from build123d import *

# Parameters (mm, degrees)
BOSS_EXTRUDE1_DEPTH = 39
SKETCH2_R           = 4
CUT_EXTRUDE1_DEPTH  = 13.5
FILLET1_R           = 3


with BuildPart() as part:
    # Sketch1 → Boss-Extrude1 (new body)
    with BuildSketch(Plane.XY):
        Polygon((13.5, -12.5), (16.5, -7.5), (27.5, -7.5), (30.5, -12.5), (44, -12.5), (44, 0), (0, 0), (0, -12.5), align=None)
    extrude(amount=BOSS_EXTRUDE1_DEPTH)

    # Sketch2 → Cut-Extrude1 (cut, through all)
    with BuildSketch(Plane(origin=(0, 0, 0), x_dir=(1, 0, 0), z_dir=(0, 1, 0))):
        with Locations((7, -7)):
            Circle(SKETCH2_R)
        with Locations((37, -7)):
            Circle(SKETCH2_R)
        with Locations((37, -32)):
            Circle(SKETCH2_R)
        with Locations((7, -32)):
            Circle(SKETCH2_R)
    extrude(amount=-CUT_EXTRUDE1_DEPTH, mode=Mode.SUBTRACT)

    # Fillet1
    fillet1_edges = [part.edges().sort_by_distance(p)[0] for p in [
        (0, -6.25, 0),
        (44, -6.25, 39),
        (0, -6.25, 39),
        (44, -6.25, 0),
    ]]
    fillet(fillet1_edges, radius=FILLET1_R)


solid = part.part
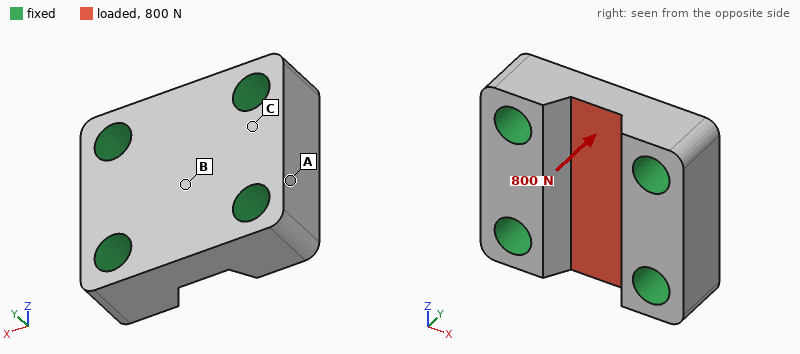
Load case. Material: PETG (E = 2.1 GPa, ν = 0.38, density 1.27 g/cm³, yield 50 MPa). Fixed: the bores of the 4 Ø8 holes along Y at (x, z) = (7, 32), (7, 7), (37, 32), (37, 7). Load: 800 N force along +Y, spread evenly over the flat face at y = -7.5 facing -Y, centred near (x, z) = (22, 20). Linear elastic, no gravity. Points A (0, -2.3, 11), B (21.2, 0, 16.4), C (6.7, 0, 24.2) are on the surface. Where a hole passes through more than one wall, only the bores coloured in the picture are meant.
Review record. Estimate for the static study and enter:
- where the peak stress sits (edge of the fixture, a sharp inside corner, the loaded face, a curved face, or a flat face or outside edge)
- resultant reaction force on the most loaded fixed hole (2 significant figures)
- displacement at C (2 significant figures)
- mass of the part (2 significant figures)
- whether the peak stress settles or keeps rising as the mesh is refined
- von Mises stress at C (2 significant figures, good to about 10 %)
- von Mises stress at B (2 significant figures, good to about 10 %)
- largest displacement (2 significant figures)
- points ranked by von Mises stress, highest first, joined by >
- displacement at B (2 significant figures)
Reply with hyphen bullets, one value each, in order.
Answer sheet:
- edge of the fixture
- 200 N
- 4.5 µm
- 20 g
- keeps rising
- 0.96 MPa
- 3.3 MPa
- 29 µm
- B > C > A
- 25 µm
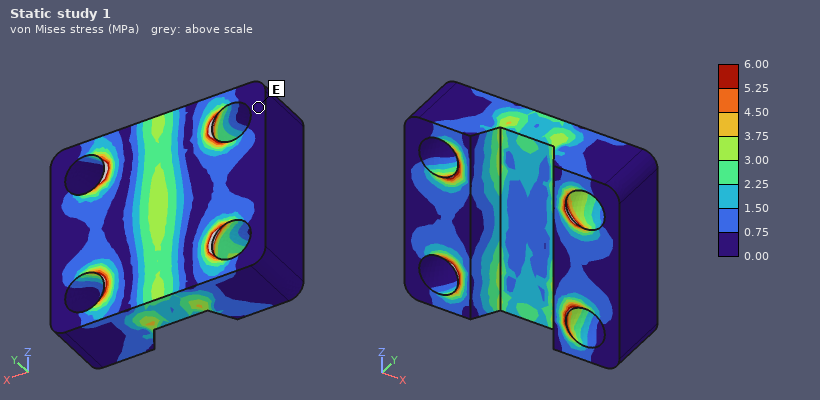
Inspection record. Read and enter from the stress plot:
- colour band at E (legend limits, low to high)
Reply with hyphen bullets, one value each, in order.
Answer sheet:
- 0.00 to 0.75 MPa
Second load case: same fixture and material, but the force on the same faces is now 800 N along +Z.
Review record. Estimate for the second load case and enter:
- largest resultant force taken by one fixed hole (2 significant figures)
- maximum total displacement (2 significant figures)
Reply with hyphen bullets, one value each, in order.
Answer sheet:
- 210 N
- 37 µm
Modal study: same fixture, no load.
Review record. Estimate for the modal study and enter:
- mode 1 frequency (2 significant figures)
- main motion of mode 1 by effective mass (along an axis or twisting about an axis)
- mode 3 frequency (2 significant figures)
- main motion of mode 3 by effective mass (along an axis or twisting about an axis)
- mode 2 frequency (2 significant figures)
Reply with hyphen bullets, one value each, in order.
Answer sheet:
- 12 kHz
- along Y
- 16 kHz
- along Z
- 15 kHz
